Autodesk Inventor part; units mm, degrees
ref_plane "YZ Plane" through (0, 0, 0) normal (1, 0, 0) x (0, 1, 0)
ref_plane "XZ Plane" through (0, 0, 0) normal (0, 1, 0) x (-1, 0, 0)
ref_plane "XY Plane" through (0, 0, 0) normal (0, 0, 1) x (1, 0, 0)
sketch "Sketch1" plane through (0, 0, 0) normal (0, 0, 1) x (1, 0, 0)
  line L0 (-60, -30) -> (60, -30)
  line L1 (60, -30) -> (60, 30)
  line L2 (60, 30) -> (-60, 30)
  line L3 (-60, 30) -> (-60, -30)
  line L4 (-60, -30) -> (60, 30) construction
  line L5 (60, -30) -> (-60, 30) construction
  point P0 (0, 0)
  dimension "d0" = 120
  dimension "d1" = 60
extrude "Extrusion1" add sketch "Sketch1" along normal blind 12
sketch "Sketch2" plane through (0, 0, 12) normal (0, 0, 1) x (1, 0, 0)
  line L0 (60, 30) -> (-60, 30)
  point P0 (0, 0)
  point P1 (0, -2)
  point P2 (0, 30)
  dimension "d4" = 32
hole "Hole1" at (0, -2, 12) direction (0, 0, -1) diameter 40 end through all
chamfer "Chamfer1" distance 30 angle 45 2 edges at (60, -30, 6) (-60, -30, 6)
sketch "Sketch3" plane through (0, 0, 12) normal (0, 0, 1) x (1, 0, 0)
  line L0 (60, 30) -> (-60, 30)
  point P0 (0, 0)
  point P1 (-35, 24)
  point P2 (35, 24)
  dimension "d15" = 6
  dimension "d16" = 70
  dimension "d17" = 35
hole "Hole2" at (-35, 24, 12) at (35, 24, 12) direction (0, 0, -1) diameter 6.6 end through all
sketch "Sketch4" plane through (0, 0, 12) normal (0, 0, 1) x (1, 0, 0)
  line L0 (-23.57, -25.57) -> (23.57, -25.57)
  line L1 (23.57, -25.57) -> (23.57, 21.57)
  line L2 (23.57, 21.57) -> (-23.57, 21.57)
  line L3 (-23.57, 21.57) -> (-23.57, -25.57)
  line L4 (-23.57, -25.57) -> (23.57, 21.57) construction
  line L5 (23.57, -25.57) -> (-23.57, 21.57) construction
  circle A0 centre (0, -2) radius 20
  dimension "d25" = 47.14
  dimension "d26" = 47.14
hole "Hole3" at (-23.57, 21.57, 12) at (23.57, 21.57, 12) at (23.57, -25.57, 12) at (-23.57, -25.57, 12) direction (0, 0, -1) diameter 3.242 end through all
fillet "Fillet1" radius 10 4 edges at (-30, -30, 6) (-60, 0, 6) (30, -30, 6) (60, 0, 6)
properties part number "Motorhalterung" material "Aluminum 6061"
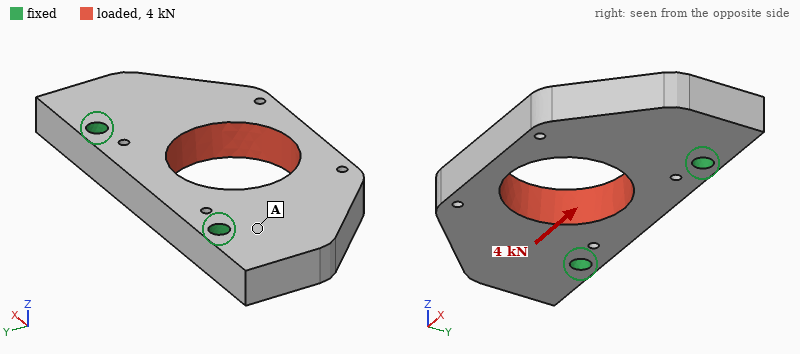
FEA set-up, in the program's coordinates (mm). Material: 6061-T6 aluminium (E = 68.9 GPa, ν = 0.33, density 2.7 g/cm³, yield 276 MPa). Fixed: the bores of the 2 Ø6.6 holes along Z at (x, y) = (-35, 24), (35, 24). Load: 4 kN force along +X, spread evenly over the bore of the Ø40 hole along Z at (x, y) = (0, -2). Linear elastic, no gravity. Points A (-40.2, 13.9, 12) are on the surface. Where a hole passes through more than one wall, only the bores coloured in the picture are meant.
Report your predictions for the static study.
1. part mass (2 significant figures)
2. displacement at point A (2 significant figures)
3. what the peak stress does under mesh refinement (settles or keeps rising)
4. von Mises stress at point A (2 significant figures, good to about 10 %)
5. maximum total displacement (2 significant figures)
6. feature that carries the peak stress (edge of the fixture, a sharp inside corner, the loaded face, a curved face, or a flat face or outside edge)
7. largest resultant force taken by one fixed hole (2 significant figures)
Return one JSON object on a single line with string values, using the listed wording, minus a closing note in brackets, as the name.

{"part mass": "160 g", "displacement at point A": "5.3 µm", "what the peak stress does under mesh refinement": "keeps rising", "von Mises stress at point A": "6.6 MPa", "maximum total displacement": "25 µm", "feature that carries the peak stress": "edge of the fixture", "largest resultant force taken by one fixed hole": "2.3 kN"}
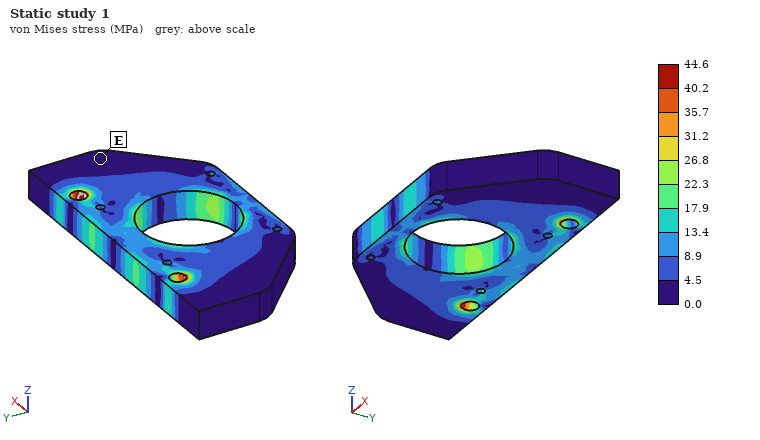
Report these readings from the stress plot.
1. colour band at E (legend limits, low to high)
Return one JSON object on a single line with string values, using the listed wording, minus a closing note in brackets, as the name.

{"colour band at E": "0.0 to 4.5 MPa"}
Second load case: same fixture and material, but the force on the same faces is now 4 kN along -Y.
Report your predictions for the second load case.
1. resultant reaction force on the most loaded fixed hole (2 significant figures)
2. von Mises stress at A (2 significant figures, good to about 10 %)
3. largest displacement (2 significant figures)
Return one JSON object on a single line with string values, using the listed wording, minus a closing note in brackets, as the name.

{"resultant reaction force on the most loaded fixed hole": "2.1 kN", "von Mises stress at A": "5.3 MPa", "largest displacement": "8.9 µm"}
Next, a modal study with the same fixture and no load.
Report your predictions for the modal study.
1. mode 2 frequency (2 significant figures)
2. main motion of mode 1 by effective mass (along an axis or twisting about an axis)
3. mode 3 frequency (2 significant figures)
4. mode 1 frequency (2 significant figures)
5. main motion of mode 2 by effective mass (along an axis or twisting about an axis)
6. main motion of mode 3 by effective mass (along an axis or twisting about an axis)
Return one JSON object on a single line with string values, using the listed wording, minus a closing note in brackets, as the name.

{"mode 2 frequency": "5100 Hz", "main motion of mode 1 by effective mass": "along Z", "mode 3 frequency": "6500 Hz", "mode 1 frequency": "3000 Hz", "main motion of mode 2 by effective mass": "twisting about Y", "main motion of mode 3 by effective mass": "along X"}
